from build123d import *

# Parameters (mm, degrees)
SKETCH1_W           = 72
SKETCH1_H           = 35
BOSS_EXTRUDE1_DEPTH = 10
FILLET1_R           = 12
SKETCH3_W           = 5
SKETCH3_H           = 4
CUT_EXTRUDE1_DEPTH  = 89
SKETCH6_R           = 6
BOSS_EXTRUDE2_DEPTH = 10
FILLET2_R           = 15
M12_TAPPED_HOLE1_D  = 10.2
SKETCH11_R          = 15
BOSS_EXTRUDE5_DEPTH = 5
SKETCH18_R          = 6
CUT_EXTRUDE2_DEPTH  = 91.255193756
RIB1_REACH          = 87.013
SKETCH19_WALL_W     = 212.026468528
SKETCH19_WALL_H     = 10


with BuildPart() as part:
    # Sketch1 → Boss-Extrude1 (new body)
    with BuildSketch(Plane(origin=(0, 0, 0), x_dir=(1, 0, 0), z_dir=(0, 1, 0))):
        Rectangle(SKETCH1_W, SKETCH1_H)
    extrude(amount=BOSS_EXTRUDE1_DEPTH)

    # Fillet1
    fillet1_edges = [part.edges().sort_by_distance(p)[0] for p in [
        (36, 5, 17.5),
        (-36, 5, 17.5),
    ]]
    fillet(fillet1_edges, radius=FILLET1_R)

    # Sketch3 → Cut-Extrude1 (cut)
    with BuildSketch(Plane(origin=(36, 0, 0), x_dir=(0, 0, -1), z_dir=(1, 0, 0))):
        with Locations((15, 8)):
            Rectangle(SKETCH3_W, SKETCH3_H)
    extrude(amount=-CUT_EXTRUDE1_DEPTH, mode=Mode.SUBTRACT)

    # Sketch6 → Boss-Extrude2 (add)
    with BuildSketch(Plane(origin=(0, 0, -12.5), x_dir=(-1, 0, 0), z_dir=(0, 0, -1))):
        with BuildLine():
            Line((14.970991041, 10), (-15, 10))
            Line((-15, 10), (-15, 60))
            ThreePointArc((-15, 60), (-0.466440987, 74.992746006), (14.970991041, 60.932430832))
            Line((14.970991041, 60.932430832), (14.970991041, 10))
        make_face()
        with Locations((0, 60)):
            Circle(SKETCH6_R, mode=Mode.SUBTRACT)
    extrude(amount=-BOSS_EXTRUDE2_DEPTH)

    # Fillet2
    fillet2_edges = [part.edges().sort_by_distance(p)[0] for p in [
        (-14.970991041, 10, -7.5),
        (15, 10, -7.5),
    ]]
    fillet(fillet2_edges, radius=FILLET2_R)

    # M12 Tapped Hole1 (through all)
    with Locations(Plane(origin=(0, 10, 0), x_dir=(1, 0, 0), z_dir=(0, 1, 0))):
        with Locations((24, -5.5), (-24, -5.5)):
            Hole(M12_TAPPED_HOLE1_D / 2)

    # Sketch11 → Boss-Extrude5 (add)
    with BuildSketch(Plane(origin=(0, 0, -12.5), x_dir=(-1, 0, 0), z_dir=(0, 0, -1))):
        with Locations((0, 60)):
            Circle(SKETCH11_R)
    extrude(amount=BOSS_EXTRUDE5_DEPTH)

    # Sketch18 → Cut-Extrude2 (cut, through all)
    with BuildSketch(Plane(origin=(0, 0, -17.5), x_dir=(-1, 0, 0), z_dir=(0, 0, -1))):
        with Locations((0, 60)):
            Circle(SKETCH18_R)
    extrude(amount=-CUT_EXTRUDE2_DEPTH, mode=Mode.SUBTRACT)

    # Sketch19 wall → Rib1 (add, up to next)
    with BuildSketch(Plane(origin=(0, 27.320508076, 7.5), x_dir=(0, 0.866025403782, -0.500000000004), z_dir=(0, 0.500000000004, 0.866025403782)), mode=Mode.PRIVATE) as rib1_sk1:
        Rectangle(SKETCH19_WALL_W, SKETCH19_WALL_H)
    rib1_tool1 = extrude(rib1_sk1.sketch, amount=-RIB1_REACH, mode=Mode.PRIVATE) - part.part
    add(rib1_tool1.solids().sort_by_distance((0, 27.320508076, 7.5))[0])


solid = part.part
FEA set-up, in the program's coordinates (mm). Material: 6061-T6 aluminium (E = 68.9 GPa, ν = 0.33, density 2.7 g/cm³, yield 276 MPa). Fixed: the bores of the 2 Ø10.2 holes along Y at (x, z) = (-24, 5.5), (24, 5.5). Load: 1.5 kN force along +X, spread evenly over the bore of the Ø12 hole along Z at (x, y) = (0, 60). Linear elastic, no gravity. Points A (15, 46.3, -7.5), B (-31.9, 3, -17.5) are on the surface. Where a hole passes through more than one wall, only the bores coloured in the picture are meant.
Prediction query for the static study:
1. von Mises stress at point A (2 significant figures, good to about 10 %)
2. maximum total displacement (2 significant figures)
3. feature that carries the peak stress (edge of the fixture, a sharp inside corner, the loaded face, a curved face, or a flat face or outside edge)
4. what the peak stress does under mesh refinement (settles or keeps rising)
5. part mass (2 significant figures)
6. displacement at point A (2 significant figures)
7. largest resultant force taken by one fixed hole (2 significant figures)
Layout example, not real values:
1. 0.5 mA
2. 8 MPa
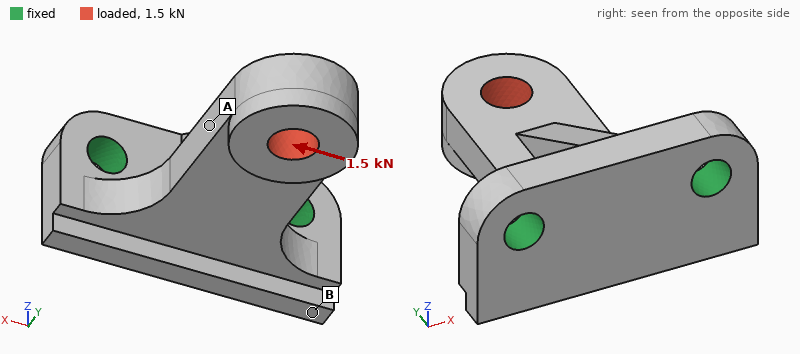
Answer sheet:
1. 14 MPa
2. 86 µm
3. edge of the fixture
4. keeps rising
5. 120 g
6. 44 µm
7. 2.1 kN
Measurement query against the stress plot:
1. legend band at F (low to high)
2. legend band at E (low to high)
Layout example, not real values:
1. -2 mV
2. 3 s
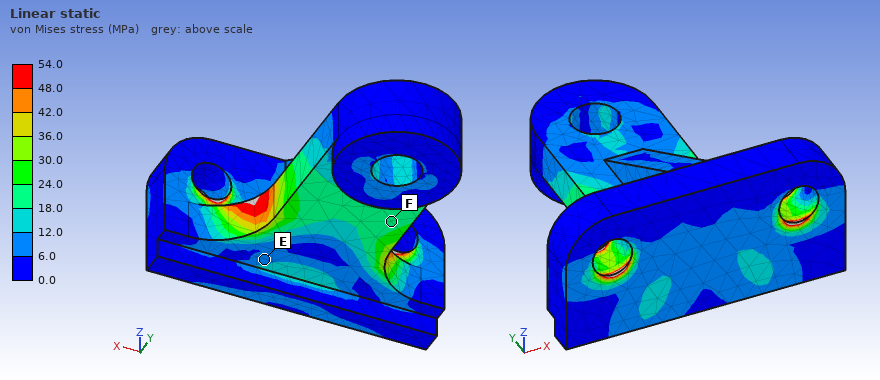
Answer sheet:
1. 18.0 to 24.0 MPa
2. 6.0 to 12.0 MPa
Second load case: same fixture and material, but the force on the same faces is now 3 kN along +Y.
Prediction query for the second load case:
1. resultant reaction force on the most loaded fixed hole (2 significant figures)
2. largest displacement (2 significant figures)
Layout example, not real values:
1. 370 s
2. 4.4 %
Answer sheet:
1. 1.6 kN
2. 0.10 mm
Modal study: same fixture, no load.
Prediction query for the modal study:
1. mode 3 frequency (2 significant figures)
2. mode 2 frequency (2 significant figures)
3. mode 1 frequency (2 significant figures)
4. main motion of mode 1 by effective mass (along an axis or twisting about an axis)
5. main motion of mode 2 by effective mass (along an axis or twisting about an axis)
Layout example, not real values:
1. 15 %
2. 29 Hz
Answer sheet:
1. 8100 Hz
2. 4500 Hz
3. 2400 Hz
4. along Z
5. along X
